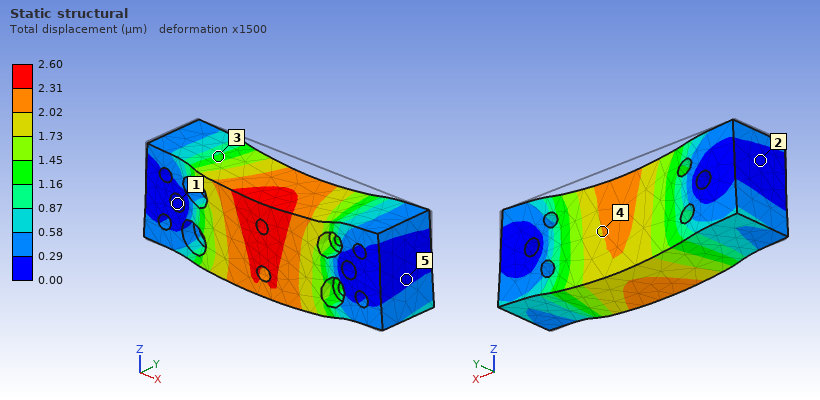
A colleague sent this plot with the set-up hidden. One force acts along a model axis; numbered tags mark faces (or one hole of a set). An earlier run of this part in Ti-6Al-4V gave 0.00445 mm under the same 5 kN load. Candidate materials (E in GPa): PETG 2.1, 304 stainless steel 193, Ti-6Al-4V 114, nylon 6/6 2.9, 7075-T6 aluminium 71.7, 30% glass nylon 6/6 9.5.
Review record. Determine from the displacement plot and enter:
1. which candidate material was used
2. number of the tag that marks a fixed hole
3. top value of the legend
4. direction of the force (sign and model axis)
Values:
304 stainless steel
1
2.60 µm
-Z
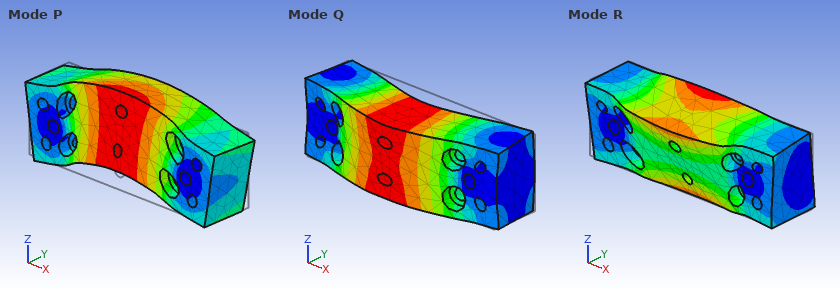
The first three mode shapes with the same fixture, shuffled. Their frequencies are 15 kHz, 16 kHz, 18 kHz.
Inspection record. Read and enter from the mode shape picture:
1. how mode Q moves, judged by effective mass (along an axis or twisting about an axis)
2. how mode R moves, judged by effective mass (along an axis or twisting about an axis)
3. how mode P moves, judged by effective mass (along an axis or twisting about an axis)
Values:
along Y
twisting about X
along Z
